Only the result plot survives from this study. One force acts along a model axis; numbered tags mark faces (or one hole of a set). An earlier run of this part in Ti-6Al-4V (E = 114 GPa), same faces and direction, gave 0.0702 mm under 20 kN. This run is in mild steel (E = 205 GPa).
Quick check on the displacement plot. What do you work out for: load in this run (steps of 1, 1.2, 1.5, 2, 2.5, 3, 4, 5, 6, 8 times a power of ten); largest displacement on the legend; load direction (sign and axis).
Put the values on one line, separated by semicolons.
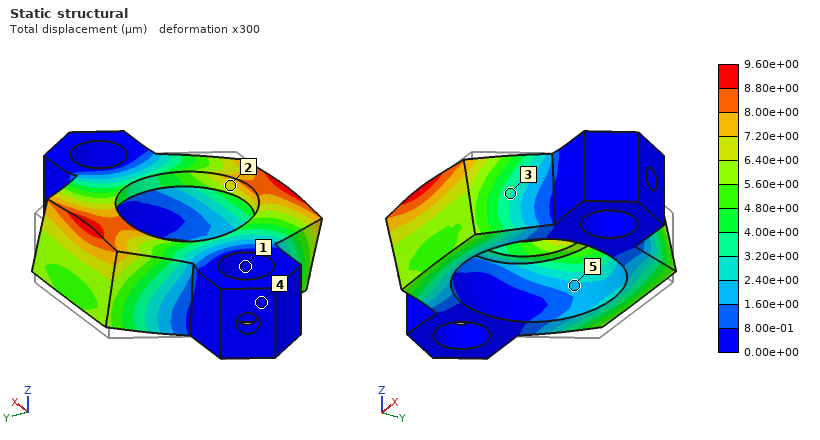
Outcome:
5 kN; 9.60e+00 µm; -Y
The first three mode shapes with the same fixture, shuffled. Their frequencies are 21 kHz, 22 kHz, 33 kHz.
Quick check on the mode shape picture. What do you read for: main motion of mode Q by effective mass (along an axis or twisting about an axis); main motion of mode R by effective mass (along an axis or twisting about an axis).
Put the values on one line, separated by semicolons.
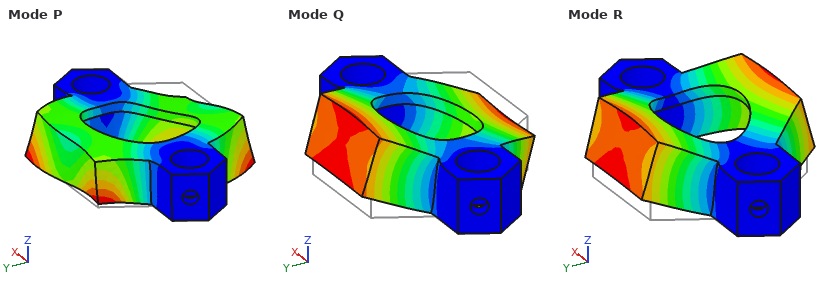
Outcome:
twisting about X; along Z
